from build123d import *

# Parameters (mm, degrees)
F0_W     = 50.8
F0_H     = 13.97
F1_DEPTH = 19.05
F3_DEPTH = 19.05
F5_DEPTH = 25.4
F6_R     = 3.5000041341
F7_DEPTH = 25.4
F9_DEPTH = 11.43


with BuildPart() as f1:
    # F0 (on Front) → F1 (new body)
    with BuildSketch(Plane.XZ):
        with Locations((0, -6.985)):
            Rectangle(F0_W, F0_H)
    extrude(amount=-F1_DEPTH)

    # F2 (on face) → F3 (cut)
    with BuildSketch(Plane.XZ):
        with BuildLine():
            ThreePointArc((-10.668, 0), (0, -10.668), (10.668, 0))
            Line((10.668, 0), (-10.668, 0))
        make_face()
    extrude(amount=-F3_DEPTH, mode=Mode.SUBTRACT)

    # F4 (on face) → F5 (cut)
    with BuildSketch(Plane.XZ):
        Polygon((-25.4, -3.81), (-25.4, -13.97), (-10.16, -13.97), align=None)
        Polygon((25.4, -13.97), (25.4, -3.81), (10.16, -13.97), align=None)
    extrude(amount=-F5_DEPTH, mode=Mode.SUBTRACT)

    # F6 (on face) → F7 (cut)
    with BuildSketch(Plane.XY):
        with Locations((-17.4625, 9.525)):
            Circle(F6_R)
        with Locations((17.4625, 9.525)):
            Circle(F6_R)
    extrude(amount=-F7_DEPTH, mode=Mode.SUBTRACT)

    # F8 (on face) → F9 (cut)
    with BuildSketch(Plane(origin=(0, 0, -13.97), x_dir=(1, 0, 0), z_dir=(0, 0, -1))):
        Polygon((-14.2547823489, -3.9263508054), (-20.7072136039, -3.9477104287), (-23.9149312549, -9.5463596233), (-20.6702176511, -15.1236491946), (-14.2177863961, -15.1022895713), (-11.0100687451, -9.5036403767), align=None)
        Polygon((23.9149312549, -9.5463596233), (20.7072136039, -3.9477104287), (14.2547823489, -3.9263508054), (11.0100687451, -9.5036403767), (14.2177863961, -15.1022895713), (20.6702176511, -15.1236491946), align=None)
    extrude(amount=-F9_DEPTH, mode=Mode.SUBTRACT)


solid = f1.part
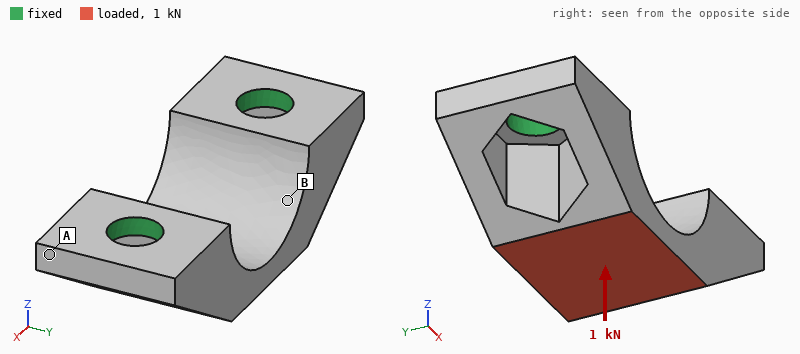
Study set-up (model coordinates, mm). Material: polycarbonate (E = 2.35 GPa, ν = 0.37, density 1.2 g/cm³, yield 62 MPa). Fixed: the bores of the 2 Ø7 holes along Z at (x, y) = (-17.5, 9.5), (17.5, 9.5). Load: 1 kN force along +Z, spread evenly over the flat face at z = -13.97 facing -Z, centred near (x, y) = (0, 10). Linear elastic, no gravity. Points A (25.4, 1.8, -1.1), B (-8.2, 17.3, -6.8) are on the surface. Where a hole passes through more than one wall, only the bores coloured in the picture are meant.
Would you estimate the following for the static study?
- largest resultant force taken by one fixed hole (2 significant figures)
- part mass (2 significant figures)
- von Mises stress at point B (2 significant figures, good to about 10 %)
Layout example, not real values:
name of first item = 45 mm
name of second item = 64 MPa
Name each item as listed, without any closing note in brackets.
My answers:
largest resultant force taken by one fixed hole = 640 N
part mass = 6.7 g
von Mises stress at point B = 12 MPa
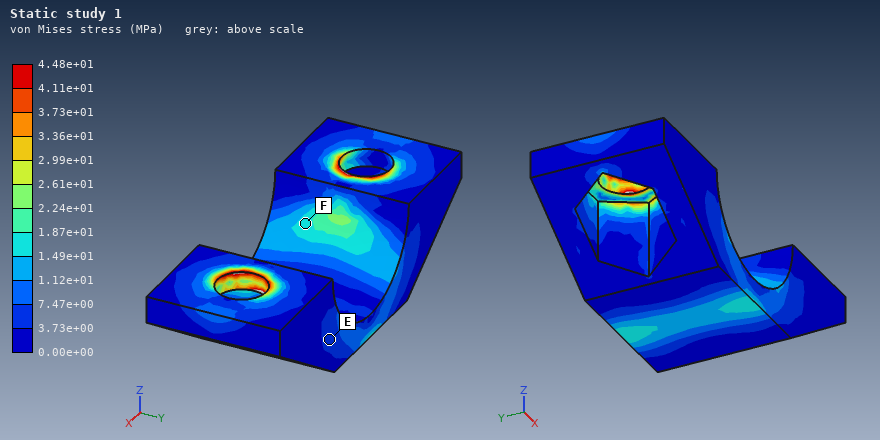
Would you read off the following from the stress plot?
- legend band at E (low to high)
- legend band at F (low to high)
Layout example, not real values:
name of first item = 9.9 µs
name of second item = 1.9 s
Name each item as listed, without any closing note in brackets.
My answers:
legend band at E = 3.73e+00 to 7.47e+00 MPa
legend band at F = 1.49e+01 to 1.87e+01 MPa
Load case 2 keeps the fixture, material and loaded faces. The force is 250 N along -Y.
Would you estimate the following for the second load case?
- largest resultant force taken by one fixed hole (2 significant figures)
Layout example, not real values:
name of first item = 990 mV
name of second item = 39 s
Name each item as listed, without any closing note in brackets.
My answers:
largest resultant force taken by one fixed hole = 130 N
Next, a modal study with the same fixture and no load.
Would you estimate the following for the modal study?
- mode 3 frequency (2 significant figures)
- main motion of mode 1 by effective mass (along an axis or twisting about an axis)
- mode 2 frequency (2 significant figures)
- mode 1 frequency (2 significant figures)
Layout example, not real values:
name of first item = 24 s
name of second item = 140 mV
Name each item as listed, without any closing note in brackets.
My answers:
mode 3 frequency = 5700 Hz
main motion of mode 1 by effective mass = along Y
mode 2 frequency = 5600 Hz
mode 1 frequency = 2900 Hz
